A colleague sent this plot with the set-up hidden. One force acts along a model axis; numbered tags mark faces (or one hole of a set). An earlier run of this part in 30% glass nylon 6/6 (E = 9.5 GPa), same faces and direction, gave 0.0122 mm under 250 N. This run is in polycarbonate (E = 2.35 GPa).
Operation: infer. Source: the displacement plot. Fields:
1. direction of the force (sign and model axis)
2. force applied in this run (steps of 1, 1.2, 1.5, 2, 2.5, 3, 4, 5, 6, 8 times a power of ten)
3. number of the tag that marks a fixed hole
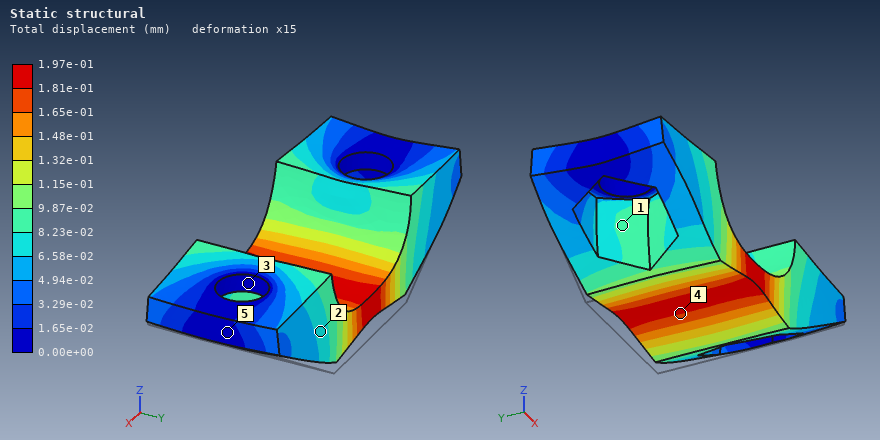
+Z
1 kN
3
